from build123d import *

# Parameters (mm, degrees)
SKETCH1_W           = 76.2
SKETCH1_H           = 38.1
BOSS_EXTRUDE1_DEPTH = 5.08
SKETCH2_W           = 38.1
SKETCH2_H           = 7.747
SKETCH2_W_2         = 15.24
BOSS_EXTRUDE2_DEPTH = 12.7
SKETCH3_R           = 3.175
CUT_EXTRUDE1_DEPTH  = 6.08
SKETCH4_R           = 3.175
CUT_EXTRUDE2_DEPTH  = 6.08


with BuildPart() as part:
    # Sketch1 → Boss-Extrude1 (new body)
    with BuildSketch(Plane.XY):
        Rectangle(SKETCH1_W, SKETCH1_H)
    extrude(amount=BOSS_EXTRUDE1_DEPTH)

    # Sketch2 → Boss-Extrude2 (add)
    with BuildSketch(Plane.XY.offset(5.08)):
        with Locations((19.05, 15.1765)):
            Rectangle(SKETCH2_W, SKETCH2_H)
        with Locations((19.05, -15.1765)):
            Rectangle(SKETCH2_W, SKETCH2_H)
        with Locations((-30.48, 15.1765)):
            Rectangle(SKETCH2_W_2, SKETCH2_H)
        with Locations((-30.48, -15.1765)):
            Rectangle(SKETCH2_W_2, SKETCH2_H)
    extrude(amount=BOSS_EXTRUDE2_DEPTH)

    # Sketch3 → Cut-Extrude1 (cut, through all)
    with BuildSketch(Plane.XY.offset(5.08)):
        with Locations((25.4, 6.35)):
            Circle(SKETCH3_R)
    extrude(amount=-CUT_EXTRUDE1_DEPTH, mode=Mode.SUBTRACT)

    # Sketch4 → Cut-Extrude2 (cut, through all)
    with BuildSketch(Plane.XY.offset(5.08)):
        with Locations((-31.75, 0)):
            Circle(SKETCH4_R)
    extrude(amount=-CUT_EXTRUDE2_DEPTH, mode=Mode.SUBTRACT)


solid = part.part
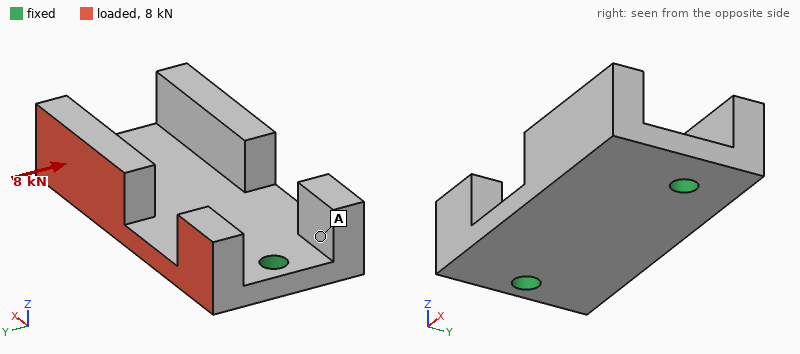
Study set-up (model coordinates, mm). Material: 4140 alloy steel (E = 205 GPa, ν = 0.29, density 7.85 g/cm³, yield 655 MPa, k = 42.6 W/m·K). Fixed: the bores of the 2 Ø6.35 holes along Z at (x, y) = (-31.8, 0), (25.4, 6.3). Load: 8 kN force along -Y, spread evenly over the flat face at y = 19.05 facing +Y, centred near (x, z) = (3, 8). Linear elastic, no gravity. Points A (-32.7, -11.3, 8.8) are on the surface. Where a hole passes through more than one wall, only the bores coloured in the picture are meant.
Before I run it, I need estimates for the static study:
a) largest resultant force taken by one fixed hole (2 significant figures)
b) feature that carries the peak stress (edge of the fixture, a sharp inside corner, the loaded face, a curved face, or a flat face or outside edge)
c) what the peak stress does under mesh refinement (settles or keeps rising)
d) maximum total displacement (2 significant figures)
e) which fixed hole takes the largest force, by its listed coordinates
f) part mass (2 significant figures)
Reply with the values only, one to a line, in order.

4.9 kN
edge of the fixture
keeps rising
70 µm
(25.4, 6.3)
200 g
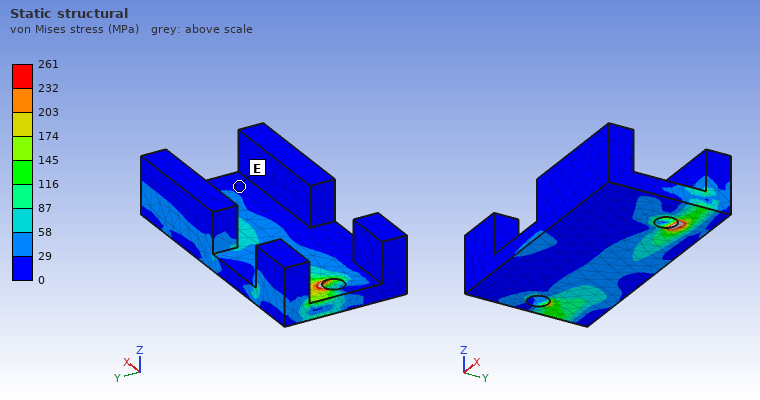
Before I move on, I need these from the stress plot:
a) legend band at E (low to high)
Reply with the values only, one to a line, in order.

0 to 29 MPa
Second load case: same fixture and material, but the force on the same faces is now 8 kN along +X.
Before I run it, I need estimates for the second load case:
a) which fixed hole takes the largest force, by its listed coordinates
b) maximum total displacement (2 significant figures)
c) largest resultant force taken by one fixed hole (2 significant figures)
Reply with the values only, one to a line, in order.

(25.4, 6.3)
25 µm
5.6 kN
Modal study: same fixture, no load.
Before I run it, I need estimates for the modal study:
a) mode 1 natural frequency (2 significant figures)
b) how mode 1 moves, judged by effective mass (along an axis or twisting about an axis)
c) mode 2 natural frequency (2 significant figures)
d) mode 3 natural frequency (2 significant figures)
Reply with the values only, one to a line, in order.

3500 Hz
along Z
5900 Hz
6000 Hz
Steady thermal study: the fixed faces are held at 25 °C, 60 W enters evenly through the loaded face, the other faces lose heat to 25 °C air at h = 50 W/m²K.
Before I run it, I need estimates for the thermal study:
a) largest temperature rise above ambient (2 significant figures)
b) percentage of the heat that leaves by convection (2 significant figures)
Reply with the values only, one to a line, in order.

66 K
19 %
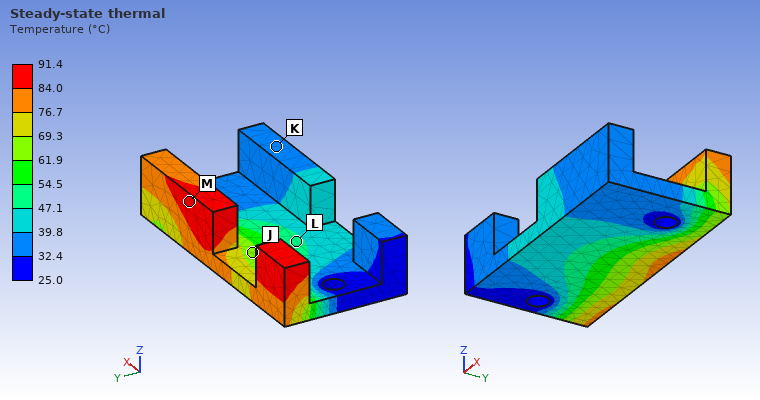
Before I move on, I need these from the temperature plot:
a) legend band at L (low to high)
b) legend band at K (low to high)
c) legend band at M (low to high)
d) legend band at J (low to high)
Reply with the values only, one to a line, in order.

47.1 to 54.5 °C
32.4 to 39.8 °C
84.0 to 91.4 °C
61.9 to 69.3 °C
